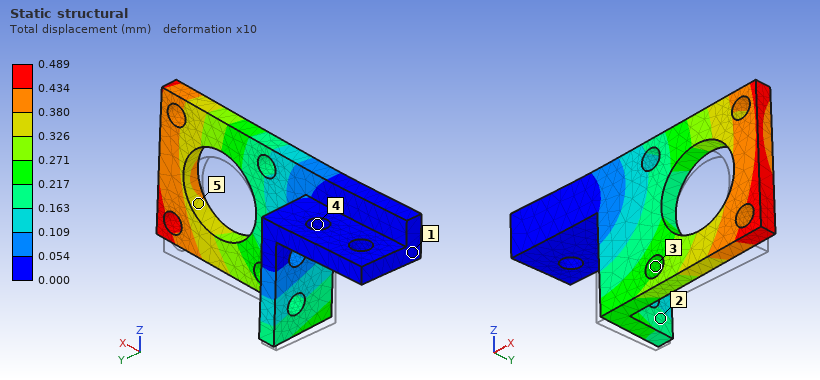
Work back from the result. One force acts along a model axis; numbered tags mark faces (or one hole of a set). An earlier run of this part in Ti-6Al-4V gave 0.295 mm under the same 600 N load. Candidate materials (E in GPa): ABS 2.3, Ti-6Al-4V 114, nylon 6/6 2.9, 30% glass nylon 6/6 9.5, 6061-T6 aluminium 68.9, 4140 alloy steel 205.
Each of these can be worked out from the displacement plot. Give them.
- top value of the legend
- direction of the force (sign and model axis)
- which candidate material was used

0.489 mm
+Z
6061-T6 aluminium
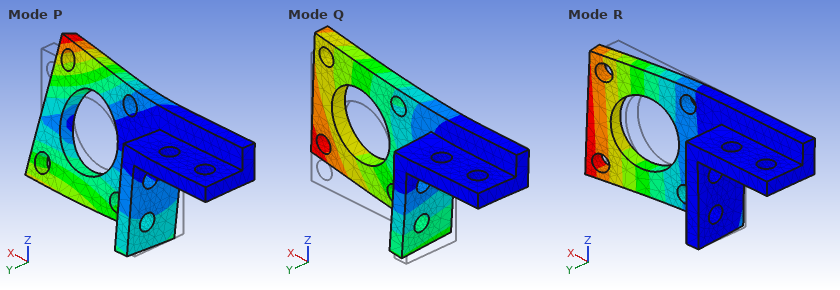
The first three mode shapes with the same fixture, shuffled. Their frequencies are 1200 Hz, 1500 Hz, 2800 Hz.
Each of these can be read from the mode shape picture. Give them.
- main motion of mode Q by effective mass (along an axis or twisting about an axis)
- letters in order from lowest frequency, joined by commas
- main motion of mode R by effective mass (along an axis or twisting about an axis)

along Z
R, Q, P
along Y
